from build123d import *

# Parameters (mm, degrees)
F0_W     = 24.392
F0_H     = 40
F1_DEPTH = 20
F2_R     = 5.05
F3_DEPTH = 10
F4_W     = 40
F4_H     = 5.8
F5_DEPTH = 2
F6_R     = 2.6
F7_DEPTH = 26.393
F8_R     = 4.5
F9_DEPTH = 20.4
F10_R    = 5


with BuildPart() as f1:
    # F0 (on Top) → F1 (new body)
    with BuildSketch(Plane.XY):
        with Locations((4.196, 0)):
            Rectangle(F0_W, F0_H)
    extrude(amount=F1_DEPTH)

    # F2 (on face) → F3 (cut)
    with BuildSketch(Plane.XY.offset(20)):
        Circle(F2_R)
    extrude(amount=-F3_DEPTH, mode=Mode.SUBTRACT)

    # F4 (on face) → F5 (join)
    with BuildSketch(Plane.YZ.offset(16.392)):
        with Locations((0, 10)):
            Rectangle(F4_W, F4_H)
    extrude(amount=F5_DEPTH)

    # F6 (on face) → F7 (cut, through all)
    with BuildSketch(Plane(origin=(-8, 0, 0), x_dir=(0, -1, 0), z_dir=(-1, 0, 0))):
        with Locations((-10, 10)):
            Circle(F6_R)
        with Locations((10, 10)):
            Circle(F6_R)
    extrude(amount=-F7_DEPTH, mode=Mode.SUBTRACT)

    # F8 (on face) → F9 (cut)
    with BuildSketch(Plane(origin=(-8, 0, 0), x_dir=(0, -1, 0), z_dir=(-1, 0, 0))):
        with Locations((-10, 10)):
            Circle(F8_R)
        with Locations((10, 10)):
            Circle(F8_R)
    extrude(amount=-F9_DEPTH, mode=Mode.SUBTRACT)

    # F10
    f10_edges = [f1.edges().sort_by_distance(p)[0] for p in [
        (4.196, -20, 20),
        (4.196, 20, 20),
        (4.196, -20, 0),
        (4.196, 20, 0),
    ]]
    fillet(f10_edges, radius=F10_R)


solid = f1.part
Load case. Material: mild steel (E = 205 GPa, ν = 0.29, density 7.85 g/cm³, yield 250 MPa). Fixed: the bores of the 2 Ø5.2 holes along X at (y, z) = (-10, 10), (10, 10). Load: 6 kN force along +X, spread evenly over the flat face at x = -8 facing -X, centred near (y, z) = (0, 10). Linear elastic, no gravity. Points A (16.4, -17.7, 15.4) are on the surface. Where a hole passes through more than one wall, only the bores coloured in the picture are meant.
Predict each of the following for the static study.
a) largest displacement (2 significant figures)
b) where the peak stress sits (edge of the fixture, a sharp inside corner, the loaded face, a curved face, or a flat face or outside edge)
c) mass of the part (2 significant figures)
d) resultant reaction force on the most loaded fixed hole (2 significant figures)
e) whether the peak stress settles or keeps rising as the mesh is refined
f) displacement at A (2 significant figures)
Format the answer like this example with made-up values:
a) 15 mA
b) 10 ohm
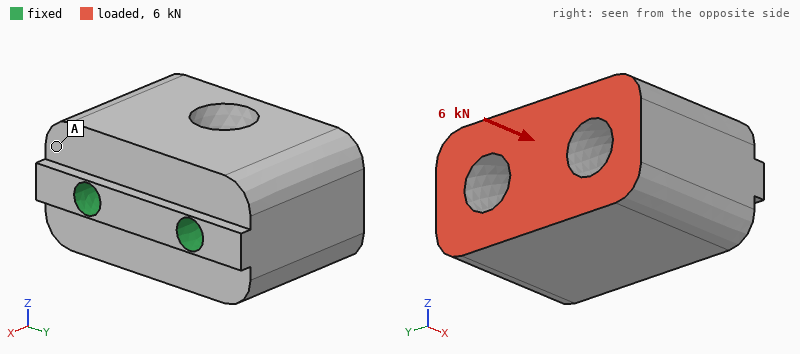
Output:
a) 4.2 µm
b) edge of the fixture
c) 120 g
d) 3.0 kN
e) keeps rising
f) 1.9 µm
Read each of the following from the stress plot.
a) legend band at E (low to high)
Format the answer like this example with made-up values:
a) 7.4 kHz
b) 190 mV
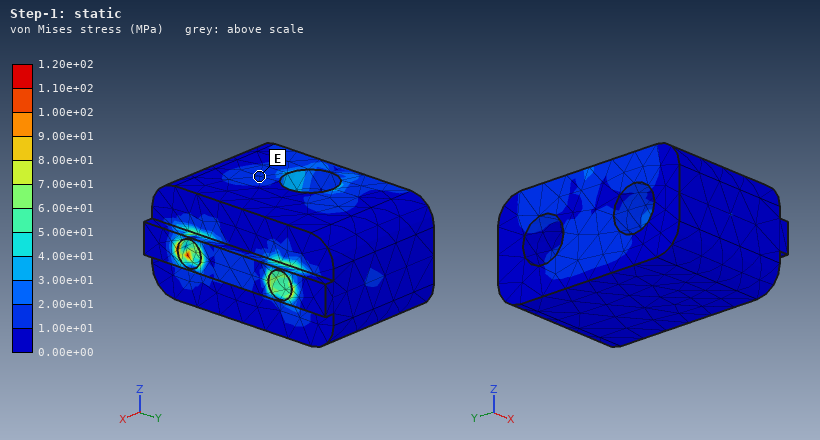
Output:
a) 1.00e+01 to 2.00e+01 MPa
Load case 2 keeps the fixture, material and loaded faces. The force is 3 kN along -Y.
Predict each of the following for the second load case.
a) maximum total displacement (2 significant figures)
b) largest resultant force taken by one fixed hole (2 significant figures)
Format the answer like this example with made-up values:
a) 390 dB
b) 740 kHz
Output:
a) 9.0 µm
b) 3.2 kN
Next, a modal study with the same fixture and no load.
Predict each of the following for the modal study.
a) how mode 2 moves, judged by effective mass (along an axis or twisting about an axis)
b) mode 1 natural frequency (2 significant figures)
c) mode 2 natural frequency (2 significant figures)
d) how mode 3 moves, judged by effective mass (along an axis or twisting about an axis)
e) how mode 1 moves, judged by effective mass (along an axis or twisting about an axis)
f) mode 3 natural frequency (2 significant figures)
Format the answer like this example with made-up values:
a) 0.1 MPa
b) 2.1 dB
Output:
a) along Y
b) 6900 Hz
c) 15 kHz
d) twisting about X
e) along Z
f) 18 kHz
